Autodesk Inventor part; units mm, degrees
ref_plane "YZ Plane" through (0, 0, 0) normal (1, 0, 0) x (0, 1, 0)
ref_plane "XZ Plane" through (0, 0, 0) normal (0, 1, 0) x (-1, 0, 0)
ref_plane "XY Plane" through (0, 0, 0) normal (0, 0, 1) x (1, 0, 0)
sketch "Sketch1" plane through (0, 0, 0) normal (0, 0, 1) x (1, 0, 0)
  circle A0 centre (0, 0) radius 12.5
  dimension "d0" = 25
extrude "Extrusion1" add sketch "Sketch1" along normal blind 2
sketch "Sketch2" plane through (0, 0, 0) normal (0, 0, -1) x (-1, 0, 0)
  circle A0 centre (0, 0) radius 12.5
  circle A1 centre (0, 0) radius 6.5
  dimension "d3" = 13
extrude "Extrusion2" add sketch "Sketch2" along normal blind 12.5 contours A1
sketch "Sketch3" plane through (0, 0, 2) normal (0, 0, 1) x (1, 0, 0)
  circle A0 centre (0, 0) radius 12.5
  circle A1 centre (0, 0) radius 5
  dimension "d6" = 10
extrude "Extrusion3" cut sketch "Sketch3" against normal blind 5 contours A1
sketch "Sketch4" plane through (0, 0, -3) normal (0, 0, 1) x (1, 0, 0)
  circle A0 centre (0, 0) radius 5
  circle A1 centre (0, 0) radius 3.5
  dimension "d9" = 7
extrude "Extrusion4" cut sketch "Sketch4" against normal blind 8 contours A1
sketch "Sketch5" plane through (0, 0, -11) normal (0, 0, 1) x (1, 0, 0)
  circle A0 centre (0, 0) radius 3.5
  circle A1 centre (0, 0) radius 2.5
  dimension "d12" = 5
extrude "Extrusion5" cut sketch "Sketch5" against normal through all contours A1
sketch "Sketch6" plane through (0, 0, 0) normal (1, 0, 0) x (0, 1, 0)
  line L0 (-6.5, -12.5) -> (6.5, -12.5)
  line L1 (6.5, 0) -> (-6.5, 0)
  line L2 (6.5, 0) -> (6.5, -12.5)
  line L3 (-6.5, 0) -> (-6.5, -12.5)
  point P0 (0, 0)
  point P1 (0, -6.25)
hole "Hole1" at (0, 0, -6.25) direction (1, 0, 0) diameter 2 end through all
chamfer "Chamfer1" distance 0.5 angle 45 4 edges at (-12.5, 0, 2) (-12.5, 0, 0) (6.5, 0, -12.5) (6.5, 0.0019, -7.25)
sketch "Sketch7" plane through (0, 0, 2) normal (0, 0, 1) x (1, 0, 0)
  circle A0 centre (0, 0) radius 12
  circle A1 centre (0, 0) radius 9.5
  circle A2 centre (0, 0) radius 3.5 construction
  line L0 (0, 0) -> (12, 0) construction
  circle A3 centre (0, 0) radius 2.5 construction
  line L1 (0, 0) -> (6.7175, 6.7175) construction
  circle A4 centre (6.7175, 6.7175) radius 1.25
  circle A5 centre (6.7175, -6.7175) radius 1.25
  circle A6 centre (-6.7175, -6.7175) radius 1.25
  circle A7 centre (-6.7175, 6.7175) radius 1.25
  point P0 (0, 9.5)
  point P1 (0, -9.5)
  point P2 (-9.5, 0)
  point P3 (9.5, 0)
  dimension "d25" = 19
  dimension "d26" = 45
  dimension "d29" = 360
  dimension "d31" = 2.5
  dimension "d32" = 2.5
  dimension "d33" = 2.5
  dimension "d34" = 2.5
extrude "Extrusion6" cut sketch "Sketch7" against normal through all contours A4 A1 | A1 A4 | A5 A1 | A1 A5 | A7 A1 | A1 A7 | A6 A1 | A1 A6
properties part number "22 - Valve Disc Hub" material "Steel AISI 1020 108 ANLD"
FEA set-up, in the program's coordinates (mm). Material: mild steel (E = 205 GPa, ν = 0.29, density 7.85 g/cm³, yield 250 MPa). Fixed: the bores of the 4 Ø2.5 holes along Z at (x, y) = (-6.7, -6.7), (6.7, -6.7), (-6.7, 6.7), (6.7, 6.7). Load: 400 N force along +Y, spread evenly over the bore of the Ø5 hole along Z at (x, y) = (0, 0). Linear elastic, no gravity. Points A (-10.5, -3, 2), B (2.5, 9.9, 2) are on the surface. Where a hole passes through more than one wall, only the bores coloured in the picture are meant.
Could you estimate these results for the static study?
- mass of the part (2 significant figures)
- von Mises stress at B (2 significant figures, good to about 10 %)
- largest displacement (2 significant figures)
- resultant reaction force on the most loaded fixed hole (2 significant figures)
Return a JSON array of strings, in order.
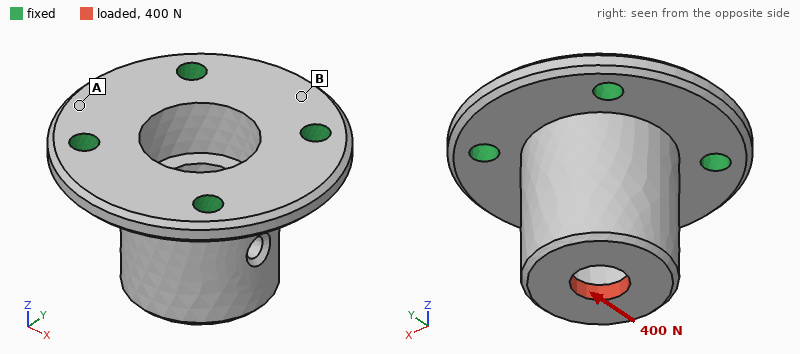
["14 g", "19 MPa", "7.4 µm", "250 N"]
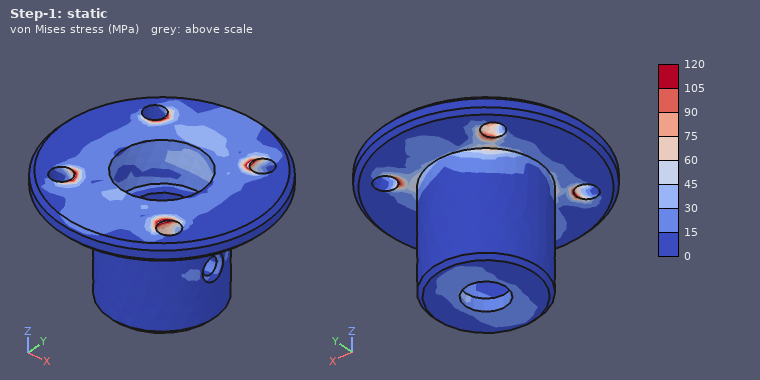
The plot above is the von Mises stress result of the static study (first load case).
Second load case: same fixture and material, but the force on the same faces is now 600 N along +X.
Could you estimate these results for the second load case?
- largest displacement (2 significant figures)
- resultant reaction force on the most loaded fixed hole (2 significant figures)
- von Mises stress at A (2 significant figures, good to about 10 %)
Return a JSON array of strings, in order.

["11 µm", "370 N", "22 MPa"]
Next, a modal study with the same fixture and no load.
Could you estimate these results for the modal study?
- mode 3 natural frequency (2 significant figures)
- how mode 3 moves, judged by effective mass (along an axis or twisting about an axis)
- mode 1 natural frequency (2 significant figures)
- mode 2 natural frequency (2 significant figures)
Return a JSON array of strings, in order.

["34 kHz", "along Z", "19 kHz", "19 kHz"]
